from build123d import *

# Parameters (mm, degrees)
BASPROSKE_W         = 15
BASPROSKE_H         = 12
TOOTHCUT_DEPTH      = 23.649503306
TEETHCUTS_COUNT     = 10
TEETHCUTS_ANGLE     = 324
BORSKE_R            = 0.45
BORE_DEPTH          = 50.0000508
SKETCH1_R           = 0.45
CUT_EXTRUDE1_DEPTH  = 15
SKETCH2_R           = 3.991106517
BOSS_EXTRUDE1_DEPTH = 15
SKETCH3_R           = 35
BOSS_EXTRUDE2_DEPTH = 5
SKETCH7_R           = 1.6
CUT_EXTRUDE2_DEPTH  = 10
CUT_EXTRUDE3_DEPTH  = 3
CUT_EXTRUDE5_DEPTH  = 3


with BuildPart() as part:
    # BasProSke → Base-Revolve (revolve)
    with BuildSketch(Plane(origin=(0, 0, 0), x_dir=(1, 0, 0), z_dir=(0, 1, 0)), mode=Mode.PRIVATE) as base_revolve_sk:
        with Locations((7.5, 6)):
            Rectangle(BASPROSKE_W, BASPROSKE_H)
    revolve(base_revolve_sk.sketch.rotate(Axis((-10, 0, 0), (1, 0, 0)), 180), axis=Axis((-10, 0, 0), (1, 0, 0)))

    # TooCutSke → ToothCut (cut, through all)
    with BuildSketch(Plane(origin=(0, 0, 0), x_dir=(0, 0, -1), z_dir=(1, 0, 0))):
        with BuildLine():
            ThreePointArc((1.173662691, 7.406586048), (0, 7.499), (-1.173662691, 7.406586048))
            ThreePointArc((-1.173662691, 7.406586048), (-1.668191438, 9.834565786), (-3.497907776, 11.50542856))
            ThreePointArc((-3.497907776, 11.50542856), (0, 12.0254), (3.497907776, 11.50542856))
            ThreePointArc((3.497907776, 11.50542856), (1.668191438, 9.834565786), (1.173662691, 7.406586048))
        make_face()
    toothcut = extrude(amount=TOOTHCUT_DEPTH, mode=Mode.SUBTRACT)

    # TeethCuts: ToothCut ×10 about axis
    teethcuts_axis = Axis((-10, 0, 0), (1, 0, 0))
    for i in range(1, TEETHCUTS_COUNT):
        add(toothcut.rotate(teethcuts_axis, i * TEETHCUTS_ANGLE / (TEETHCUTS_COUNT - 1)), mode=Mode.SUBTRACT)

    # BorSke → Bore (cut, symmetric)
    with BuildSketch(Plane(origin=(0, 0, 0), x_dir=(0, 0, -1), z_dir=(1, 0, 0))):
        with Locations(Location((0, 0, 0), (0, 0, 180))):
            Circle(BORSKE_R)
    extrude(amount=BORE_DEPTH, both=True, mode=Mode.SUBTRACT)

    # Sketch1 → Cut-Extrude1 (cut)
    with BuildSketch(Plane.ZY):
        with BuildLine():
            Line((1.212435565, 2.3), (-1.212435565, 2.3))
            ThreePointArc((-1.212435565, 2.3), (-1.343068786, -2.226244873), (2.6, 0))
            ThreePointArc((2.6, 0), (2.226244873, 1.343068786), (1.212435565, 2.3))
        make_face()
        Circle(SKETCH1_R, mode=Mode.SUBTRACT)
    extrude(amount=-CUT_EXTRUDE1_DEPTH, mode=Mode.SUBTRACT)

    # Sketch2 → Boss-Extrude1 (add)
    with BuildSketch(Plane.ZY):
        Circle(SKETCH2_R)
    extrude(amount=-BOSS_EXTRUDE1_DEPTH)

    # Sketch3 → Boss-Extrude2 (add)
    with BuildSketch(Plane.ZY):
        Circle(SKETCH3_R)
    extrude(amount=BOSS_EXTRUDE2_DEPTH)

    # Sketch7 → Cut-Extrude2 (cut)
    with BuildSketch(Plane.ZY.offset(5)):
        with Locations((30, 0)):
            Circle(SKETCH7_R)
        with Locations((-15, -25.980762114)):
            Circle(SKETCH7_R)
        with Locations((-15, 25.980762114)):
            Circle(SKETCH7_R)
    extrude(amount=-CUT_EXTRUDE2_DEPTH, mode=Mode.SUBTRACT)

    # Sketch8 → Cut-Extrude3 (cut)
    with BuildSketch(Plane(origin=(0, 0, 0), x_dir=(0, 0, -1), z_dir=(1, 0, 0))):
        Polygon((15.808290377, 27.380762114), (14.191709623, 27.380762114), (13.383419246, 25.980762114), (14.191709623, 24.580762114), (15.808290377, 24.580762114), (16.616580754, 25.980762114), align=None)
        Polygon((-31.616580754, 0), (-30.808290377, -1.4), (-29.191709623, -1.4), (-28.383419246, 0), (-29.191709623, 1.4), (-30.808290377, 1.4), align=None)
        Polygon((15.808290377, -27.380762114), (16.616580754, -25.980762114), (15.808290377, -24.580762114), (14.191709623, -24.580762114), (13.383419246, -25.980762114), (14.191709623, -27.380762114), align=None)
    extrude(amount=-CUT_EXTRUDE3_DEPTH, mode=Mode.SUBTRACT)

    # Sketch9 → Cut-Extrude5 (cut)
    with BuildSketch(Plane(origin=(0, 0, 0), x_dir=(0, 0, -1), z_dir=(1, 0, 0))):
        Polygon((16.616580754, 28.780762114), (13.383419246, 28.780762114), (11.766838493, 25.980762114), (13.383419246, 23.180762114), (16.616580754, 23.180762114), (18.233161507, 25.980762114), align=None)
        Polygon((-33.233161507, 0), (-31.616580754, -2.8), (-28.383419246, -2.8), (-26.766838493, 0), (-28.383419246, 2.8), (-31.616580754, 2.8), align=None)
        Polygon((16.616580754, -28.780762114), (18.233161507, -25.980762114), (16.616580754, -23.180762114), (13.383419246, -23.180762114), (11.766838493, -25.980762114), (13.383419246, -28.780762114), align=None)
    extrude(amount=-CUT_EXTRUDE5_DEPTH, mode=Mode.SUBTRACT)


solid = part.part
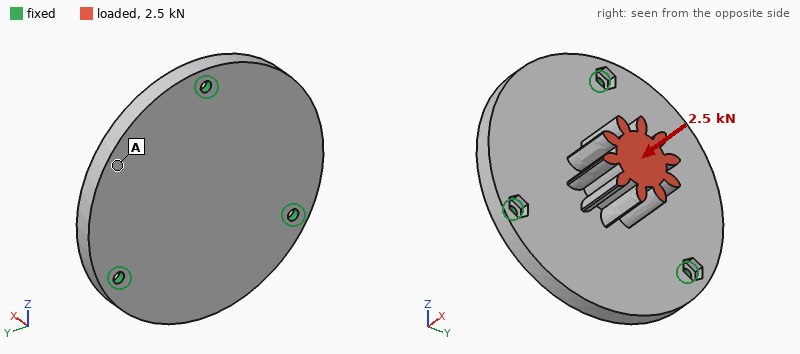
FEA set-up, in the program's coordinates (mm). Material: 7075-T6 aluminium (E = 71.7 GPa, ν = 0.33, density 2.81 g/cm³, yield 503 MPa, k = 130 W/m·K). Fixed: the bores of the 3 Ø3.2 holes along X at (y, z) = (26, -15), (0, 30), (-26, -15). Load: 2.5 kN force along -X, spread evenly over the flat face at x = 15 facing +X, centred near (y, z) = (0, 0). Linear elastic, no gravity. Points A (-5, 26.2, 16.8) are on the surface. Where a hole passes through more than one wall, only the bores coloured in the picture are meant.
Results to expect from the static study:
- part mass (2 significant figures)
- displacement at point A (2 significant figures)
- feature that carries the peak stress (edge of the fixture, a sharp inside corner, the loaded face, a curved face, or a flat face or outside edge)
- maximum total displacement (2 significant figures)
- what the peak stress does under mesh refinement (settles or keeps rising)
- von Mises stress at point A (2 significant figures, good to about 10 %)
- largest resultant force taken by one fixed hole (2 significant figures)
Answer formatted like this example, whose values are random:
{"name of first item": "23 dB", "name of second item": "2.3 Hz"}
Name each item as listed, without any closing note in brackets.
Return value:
{"part mass": "65 g", "displacement at point A": "35 µm", "feature that carries the peak stress": "edge of the fixture", "maximum total displacement": "69 µm", "what the peak stress does under mesh refinement": "keeps rising", "von Mises stress at point A": "29 MPa", "largest resultant force taken by one fixed hole": "1.4 kN"}
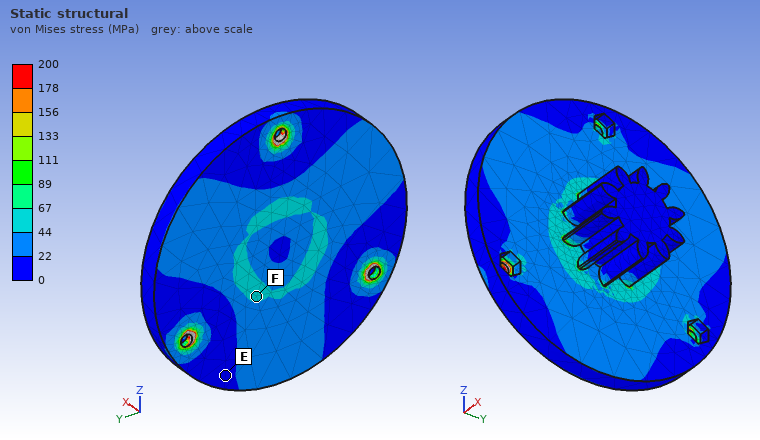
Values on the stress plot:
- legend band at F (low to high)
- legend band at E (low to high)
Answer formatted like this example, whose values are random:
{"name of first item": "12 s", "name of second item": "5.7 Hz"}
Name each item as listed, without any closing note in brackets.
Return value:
{"legend band at F": "44 to 67 MPa", "legend band at E": "0 to 22 MPa"}
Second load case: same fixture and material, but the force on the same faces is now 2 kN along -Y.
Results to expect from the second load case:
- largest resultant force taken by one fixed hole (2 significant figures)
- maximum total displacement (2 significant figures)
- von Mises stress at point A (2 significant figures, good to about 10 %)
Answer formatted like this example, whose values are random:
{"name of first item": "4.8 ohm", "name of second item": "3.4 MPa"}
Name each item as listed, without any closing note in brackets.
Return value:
{"largest resultant force taken by one fixed hole": "1.4 kN", "maximum total displacement": "81 µm", "von Mises stress at point A": "22 MPa"}
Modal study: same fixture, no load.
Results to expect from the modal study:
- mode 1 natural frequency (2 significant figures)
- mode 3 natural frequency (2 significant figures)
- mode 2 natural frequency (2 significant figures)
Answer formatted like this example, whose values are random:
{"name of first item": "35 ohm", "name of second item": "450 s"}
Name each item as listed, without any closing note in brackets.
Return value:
{"mode 1 natural frequency": "5000 Hz", "mode 3 natural frequency": "5000 Hz", "mode 2 natural frequency": "5000 Hz"}
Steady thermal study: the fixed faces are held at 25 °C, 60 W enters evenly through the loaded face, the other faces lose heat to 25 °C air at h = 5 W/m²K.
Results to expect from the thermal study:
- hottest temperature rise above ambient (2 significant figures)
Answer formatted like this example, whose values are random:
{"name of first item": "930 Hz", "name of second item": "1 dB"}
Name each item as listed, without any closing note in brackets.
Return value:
{"hottest temperature rise above ambient": "62 K"}
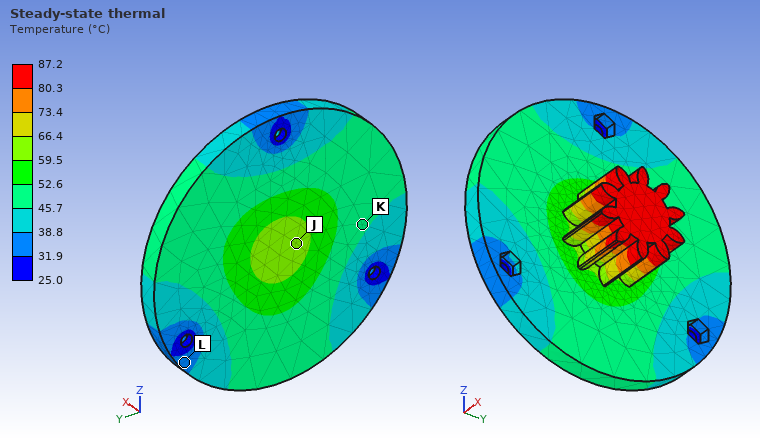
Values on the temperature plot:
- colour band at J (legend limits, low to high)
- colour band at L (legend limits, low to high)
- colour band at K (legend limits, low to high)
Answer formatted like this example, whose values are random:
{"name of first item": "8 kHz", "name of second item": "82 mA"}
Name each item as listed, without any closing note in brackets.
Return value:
{"colour band at J": "59.5 to 66.4 °C", "colour band at L": "31.9 to 38.8 °C", "colour band at K": "45.7 to 52.6 °C"}
